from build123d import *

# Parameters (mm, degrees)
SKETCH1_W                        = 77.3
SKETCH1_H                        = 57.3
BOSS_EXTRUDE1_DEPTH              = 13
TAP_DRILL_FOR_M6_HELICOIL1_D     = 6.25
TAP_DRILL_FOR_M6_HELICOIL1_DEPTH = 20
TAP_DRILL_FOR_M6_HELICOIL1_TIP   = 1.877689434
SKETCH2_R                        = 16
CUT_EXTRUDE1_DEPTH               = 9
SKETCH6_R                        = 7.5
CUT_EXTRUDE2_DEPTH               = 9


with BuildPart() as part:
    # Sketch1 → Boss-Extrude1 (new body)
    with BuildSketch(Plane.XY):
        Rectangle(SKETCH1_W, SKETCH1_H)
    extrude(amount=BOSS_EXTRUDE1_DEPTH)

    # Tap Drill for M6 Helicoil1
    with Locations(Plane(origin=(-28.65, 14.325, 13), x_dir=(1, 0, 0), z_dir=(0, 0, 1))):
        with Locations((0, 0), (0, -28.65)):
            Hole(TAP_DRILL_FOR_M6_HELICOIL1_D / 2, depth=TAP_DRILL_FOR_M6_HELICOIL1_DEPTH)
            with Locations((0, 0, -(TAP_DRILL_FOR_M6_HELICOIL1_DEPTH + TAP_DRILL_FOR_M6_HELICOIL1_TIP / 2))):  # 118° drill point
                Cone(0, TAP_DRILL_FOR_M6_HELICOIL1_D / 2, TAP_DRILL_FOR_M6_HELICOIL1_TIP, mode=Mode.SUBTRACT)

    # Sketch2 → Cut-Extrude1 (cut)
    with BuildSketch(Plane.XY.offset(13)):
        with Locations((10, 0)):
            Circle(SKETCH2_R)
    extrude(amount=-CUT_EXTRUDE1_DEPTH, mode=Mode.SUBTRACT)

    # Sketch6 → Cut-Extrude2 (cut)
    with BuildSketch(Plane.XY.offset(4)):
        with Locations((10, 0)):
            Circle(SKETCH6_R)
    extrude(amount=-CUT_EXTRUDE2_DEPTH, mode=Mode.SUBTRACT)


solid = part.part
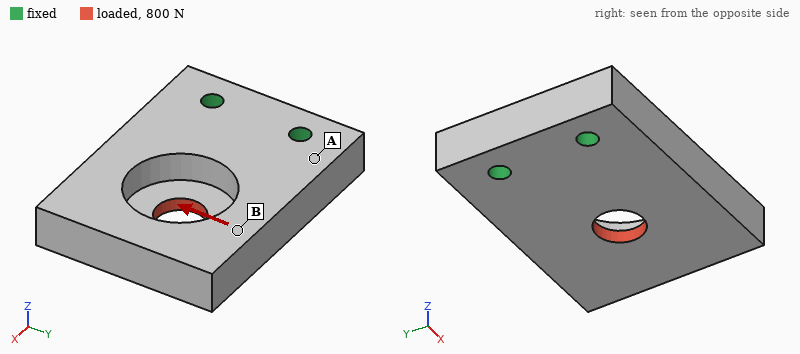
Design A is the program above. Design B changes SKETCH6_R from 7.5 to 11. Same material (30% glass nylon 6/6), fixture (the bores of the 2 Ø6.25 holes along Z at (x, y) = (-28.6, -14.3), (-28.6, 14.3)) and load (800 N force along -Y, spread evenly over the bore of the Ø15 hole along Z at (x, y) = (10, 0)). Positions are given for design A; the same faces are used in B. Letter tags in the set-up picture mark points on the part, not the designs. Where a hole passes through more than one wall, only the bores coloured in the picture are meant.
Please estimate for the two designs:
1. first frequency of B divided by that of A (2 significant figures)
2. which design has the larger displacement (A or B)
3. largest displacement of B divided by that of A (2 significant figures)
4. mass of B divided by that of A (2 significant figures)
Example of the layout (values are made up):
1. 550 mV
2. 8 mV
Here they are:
1. 1.00
2. B
3. 1.1
4. 0.98
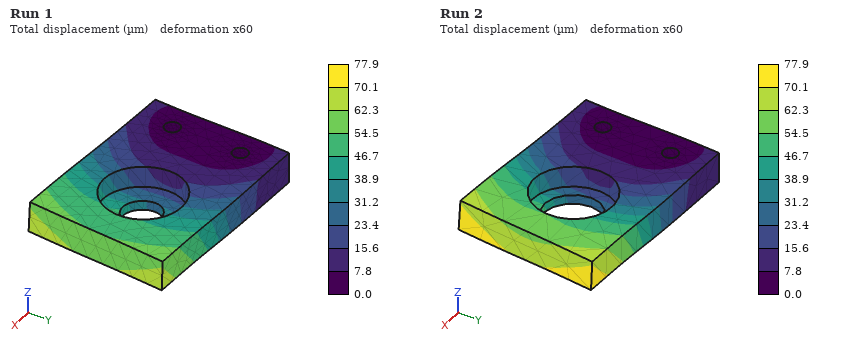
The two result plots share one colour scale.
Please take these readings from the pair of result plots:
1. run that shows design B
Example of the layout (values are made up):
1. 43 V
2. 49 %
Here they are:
1. Run 2
